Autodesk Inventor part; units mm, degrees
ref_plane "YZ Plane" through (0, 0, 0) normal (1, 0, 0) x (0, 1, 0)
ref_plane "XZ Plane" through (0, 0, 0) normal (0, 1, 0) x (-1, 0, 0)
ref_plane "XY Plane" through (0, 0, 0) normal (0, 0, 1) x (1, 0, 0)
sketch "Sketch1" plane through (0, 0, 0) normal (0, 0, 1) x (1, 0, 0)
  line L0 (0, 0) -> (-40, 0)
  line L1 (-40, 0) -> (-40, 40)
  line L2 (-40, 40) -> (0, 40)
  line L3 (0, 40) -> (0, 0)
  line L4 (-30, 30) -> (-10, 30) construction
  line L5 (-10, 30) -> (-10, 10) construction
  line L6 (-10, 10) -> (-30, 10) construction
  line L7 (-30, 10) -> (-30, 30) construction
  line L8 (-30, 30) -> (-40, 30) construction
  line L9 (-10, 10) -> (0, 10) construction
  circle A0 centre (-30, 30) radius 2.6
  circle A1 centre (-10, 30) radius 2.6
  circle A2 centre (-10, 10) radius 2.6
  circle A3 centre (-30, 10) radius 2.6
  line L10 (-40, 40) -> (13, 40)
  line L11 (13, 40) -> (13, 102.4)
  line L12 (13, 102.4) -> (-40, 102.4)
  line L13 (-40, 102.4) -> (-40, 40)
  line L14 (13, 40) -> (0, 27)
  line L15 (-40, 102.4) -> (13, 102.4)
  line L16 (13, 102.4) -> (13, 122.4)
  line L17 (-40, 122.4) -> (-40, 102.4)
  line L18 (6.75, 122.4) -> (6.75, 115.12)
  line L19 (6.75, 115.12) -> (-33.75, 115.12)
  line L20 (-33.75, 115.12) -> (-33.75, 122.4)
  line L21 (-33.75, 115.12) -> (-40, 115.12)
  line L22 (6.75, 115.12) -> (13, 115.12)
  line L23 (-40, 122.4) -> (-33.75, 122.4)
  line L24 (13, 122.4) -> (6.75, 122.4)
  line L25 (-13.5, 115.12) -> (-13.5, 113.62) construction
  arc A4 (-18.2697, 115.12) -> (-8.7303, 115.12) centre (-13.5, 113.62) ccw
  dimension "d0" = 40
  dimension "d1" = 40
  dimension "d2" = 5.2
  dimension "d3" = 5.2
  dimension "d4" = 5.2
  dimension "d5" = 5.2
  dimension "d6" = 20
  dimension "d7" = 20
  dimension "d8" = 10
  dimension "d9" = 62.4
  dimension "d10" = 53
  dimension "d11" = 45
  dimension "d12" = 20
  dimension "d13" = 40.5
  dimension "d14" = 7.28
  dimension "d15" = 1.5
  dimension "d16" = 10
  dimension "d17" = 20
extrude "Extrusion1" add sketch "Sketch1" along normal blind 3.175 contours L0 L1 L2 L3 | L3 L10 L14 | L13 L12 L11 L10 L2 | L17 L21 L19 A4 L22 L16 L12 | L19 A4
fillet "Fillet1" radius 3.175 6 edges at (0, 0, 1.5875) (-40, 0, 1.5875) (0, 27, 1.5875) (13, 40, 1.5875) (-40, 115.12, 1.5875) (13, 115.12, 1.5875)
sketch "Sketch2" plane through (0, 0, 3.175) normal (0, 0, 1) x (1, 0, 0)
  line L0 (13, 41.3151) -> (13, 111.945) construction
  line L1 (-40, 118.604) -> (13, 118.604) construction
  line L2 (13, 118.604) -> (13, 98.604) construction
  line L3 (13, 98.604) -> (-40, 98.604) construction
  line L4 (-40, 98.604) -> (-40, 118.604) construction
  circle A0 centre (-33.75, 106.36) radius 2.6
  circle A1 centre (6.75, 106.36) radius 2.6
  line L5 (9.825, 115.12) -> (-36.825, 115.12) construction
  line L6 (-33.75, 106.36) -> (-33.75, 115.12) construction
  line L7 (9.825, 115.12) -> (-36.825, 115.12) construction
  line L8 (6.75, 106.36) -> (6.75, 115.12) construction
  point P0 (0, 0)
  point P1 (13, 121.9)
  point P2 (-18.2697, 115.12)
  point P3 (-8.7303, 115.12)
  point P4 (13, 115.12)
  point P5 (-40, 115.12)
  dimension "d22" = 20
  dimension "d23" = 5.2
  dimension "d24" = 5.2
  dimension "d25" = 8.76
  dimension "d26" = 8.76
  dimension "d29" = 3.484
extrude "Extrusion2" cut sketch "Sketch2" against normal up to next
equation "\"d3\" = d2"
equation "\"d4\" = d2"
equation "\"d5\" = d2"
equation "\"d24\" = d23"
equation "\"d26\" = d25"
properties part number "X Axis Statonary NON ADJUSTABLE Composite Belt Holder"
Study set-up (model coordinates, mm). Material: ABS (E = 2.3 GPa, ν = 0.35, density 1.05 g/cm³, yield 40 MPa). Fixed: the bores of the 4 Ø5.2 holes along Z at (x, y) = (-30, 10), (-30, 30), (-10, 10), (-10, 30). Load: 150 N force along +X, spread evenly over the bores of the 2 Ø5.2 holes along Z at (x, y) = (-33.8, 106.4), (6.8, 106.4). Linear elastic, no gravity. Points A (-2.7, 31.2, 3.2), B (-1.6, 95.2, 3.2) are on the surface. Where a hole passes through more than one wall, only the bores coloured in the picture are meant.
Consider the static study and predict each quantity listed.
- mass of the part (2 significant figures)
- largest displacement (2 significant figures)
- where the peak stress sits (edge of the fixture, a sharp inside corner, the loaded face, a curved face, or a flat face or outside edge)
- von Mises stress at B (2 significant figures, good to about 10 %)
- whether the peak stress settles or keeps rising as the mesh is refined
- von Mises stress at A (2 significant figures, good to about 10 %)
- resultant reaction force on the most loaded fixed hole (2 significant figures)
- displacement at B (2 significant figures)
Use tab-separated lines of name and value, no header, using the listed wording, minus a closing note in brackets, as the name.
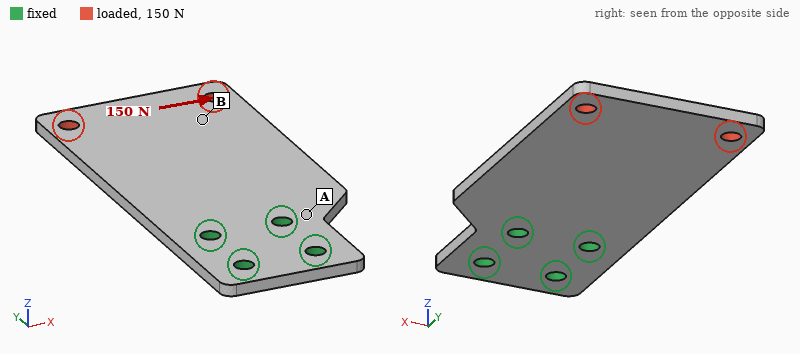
mass of the part	18 g
largest displacement	0.69 mm
where the peak stress sits	edge of the fixture
von Mises stress at B	2.0 MPa
whether the peak stress settles or keeps rising as the mesh is refined	keeps rising
von Mises stress at A	6.6 MPa
resultant reaction force on the most loaded fixed hole	390 N
displacement at B	0.50 mm
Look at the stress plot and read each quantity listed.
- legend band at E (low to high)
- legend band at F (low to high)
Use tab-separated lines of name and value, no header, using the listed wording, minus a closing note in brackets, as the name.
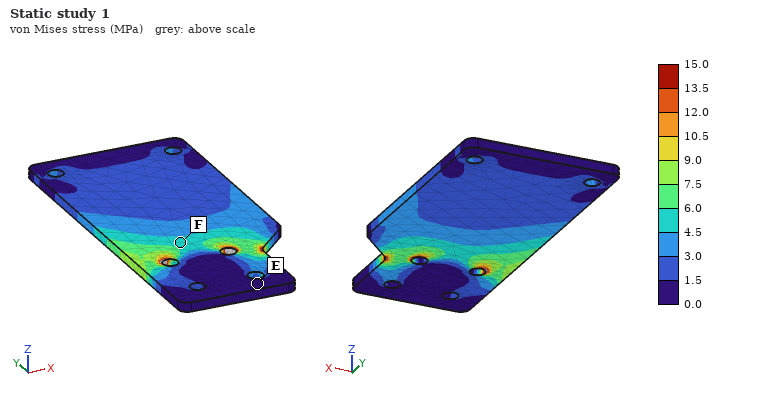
legend band at E	0.0 to 1.5 MPa
legend band at F	4.5 to 6.0 MPa
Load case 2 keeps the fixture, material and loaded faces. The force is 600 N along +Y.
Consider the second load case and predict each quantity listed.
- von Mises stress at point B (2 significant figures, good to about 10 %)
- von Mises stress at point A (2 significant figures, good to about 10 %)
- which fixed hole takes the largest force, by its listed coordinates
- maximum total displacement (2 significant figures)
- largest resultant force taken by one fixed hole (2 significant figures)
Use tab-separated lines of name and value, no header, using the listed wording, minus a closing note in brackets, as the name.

von Mises stress at point B	3.5 MPa
von Mises stress at point A	5.0 MPa
which fixed hole takes the largest force, by its listed coordinates	(-10, 30)
maximum total displacement	0.27 mm
largest resultant force taken by one fixed hole	360 N
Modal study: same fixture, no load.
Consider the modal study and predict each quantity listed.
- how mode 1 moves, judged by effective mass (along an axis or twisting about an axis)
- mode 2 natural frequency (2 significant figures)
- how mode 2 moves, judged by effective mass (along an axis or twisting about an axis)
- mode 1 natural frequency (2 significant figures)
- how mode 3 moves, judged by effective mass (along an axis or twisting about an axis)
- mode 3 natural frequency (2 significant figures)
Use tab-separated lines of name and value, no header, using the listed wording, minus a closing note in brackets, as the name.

how mode 1 moves, judged by effective mass	along Z
mode 2 natural frequency	350 Hz
how mode 2 moves, judged by effective mass	twisting about Y
mode 1 natural frequency	110 Hz
how mode 3 moves, judged by effective mass	along Z
mode 3 natural frequency	650 Hz
